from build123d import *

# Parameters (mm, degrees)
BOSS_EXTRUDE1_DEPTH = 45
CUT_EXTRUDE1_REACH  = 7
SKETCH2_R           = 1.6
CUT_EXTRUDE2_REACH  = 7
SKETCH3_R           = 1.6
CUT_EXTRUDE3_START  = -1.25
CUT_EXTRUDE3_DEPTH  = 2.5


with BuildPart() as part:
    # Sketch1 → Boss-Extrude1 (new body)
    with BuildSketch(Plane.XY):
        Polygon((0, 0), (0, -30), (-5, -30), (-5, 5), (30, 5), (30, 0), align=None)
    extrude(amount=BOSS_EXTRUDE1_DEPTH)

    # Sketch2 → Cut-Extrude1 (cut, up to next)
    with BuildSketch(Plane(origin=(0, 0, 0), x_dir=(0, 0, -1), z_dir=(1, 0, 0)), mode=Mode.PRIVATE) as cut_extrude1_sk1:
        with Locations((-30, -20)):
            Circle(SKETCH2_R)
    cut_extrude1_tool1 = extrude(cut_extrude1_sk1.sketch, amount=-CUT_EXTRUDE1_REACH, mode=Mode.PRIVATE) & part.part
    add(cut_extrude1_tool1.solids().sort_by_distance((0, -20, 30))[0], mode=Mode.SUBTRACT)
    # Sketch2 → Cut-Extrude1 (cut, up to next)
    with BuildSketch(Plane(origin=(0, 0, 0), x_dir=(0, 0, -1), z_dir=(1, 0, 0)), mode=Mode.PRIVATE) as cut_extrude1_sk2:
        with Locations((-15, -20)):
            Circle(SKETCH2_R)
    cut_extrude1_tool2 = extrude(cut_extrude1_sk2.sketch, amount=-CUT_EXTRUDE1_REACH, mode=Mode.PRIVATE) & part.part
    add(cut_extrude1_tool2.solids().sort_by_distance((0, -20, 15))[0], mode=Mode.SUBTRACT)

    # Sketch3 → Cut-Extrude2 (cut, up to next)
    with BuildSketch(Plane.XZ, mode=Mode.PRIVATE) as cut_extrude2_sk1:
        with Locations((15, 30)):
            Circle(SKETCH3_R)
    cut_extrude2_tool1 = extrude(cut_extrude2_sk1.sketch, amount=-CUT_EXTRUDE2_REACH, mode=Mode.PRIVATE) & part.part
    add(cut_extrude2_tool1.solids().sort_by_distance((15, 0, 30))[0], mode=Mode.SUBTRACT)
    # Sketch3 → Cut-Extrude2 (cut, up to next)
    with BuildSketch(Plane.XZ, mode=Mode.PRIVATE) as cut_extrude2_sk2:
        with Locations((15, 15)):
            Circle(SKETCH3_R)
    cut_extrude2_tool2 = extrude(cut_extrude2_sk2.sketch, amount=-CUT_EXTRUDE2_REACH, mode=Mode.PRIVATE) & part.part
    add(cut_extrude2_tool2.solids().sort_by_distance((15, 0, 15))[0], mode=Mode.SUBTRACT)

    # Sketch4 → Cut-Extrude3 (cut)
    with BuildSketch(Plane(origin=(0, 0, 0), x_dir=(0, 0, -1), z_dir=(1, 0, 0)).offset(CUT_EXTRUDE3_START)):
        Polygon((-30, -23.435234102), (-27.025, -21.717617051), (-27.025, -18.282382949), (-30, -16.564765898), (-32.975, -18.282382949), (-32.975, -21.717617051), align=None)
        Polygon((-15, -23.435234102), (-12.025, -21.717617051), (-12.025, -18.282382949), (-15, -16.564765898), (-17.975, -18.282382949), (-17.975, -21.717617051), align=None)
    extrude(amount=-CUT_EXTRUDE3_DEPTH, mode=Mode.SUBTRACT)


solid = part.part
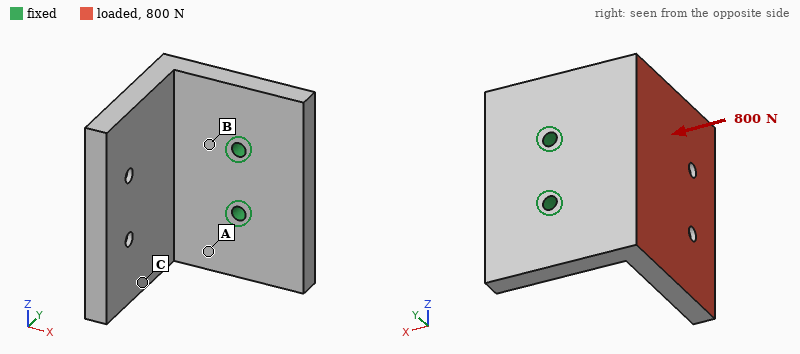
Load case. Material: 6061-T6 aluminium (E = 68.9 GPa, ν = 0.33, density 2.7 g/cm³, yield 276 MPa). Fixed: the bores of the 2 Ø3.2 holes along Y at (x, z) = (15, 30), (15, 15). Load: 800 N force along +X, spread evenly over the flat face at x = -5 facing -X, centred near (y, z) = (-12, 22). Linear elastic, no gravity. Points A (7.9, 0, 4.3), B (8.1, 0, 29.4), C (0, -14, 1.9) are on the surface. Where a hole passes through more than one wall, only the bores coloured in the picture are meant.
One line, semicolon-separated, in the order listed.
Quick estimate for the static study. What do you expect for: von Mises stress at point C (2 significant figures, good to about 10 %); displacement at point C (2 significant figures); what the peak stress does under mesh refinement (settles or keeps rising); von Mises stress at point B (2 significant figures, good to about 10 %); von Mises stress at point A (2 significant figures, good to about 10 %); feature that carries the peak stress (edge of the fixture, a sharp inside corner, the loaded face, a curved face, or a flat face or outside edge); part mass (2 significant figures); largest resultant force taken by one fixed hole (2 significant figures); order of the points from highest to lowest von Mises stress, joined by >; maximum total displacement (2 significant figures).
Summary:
16 MPa; 0.14 mm; keeps rising; 71 MPa; 54 MPa; edge of the fixture; 39 g; 400 N; B > A > C; 0.31 mm
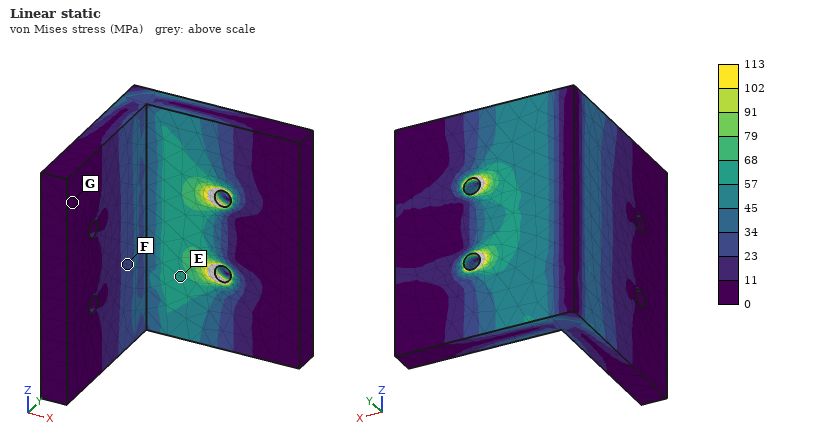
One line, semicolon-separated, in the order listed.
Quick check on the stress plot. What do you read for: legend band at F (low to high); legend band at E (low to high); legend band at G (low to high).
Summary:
23 to 34 MPa; 57 to 68 MPa; 0 to 11 MPa
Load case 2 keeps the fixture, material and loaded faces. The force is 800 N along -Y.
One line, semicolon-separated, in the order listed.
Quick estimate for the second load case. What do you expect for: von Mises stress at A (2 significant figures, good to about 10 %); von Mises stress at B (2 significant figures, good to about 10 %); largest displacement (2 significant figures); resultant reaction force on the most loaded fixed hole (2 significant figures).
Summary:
40 MPa; 61 MPa; 0.22 mm; 400 N
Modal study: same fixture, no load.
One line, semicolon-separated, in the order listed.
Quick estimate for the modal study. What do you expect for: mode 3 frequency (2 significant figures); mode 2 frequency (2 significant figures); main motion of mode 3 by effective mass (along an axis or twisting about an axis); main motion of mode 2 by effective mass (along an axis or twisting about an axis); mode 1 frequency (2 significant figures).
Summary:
6100 Hz; 3300 Hz; along Y; along Z; 2000 Hz
